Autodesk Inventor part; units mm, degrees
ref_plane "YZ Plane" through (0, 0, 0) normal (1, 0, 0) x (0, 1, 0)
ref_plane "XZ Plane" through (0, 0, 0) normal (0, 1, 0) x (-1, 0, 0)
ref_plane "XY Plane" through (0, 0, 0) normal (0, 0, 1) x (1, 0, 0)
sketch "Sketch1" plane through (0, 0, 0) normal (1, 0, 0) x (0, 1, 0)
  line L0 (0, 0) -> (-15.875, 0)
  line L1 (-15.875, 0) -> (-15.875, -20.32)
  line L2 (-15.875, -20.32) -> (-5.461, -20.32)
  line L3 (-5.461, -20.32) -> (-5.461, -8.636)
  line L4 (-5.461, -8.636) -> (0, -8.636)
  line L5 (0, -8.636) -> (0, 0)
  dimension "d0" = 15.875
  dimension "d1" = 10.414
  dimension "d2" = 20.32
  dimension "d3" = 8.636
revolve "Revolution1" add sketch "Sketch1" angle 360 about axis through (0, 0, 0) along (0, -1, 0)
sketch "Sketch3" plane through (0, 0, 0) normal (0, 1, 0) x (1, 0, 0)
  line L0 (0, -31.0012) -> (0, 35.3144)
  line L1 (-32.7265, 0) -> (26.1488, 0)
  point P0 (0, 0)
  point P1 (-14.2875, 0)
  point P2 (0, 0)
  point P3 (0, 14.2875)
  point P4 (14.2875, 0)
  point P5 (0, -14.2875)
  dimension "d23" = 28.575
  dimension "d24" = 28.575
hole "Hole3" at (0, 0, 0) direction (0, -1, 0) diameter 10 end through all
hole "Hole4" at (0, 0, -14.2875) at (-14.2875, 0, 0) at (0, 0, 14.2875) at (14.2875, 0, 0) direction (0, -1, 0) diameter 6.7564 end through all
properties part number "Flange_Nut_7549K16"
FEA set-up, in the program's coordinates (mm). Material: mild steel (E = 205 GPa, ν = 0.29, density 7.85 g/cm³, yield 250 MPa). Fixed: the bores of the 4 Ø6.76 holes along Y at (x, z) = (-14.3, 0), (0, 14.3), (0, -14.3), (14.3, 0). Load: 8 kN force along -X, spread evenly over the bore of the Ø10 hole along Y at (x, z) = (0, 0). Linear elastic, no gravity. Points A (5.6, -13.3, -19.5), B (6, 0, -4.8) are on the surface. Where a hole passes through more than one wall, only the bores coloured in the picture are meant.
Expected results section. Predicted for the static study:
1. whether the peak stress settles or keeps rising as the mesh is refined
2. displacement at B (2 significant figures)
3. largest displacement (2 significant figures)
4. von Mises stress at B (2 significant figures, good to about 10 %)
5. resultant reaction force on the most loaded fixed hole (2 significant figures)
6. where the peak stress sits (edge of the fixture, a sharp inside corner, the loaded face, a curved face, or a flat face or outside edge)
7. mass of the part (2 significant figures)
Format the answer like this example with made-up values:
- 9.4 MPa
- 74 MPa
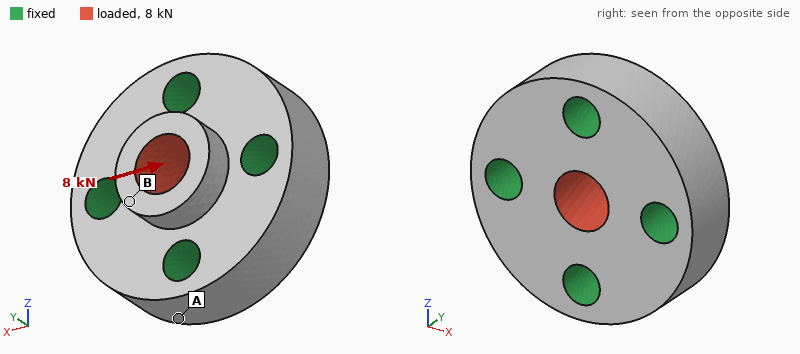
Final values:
- keeps rising
- 2.6 µm
- 3.2 µm
- 24 MPa
- 2.7 kN
- a sharp inside corner
- 95 g
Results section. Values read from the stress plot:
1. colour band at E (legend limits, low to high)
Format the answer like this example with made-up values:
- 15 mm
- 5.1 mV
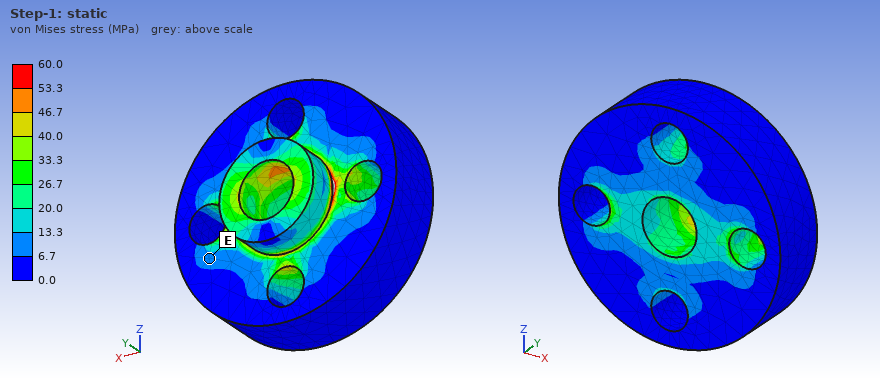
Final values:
- 6.7 to 13.3 MPa
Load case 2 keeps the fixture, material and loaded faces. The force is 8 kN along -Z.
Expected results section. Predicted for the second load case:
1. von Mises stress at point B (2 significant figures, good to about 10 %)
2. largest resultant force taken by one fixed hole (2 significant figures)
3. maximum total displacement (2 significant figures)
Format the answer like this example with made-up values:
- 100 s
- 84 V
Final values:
- 20 MPa
- 2.7 kN
- 3.2 µm
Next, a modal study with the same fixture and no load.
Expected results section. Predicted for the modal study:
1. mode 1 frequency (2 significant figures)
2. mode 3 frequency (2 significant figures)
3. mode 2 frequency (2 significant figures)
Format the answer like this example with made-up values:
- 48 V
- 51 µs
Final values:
- 62 kHz
- 63 kHz
- 63 kHz
